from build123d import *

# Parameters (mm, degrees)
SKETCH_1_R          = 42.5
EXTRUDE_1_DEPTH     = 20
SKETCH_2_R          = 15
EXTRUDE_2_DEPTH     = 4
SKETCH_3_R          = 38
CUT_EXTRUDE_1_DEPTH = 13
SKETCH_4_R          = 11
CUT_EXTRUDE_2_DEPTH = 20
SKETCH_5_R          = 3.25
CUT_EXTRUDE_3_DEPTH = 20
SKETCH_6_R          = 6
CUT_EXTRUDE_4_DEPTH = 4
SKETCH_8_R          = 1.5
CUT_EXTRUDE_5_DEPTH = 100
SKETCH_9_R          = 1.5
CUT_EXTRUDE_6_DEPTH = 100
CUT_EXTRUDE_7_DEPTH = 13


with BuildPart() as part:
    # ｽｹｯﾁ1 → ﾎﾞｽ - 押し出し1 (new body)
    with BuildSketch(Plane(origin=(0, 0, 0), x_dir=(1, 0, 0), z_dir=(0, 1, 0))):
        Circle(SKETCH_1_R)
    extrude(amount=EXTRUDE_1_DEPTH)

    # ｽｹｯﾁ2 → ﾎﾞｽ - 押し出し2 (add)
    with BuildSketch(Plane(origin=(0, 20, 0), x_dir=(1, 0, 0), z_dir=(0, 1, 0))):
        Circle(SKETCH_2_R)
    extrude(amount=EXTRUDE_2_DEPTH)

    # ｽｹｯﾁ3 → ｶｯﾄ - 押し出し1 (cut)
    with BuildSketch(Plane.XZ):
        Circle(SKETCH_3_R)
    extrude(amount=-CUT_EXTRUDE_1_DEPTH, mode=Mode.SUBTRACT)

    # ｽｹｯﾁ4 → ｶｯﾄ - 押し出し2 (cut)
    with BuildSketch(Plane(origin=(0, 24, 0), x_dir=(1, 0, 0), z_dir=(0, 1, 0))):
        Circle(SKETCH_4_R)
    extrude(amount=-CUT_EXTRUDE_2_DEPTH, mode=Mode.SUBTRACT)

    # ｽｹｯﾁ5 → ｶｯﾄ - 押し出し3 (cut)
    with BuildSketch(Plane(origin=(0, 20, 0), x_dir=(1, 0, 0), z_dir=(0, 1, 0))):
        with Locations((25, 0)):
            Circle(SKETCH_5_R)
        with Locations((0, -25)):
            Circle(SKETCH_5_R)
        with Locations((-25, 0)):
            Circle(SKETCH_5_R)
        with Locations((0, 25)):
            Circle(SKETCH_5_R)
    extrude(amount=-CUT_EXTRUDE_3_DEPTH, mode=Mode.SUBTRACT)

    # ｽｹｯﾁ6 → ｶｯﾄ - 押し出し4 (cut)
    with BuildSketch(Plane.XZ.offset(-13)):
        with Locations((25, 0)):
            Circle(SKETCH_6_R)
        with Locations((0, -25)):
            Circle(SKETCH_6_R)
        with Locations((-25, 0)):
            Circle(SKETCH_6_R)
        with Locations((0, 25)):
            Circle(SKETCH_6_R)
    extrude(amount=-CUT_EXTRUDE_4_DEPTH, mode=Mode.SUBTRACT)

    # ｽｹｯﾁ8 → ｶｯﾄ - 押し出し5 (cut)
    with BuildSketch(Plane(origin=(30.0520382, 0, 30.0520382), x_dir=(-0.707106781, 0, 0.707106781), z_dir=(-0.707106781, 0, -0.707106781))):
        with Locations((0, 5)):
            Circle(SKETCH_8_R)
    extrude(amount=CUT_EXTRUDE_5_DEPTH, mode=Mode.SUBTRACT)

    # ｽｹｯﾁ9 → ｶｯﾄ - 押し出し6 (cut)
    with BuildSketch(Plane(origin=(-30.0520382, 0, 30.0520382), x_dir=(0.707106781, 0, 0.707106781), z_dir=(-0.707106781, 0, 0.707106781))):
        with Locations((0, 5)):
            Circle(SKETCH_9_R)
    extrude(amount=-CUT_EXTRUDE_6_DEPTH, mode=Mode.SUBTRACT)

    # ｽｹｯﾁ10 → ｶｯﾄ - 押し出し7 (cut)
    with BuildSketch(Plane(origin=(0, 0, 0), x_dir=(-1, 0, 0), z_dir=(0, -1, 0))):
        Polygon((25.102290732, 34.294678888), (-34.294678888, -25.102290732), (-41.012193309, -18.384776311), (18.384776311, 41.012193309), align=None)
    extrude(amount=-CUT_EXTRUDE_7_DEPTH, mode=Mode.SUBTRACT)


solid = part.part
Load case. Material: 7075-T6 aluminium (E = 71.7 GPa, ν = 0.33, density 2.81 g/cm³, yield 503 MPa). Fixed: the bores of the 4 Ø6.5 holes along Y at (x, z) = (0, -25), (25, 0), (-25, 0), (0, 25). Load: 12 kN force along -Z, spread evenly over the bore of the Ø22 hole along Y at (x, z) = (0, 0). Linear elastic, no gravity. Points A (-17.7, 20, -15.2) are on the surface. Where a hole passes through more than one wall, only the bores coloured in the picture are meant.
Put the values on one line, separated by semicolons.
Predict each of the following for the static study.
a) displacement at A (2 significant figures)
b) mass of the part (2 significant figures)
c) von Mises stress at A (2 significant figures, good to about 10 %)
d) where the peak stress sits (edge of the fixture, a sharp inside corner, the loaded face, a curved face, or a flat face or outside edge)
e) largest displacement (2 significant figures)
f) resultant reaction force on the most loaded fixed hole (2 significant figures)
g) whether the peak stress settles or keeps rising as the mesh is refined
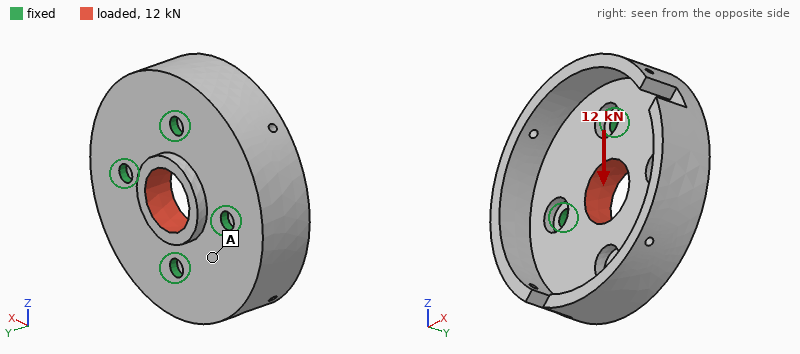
4.8 µm; 140 g; 13 MPa; edge of the fixture; 13 µm; 3.4 kN; keeps rising
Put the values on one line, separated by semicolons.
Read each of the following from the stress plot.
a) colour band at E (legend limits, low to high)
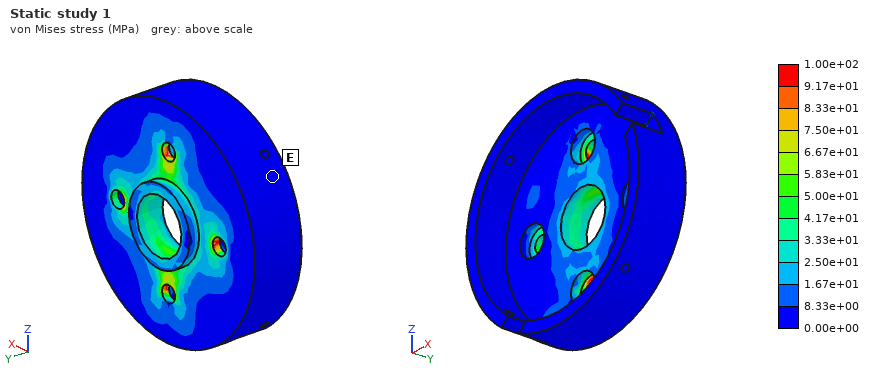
0.00e+00 to 8.33e+00 MPa
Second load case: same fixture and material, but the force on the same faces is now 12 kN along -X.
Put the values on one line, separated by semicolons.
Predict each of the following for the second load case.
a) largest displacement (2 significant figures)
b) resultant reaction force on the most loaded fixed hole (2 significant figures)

13 µm; 3.4 kN
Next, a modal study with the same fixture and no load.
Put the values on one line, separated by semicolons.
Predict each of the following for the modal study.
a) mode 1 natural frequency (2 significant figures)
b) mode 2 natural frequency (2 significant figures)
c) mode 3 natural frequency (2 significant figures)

4900 Hz; 6100 Hz; 6400 Hz
